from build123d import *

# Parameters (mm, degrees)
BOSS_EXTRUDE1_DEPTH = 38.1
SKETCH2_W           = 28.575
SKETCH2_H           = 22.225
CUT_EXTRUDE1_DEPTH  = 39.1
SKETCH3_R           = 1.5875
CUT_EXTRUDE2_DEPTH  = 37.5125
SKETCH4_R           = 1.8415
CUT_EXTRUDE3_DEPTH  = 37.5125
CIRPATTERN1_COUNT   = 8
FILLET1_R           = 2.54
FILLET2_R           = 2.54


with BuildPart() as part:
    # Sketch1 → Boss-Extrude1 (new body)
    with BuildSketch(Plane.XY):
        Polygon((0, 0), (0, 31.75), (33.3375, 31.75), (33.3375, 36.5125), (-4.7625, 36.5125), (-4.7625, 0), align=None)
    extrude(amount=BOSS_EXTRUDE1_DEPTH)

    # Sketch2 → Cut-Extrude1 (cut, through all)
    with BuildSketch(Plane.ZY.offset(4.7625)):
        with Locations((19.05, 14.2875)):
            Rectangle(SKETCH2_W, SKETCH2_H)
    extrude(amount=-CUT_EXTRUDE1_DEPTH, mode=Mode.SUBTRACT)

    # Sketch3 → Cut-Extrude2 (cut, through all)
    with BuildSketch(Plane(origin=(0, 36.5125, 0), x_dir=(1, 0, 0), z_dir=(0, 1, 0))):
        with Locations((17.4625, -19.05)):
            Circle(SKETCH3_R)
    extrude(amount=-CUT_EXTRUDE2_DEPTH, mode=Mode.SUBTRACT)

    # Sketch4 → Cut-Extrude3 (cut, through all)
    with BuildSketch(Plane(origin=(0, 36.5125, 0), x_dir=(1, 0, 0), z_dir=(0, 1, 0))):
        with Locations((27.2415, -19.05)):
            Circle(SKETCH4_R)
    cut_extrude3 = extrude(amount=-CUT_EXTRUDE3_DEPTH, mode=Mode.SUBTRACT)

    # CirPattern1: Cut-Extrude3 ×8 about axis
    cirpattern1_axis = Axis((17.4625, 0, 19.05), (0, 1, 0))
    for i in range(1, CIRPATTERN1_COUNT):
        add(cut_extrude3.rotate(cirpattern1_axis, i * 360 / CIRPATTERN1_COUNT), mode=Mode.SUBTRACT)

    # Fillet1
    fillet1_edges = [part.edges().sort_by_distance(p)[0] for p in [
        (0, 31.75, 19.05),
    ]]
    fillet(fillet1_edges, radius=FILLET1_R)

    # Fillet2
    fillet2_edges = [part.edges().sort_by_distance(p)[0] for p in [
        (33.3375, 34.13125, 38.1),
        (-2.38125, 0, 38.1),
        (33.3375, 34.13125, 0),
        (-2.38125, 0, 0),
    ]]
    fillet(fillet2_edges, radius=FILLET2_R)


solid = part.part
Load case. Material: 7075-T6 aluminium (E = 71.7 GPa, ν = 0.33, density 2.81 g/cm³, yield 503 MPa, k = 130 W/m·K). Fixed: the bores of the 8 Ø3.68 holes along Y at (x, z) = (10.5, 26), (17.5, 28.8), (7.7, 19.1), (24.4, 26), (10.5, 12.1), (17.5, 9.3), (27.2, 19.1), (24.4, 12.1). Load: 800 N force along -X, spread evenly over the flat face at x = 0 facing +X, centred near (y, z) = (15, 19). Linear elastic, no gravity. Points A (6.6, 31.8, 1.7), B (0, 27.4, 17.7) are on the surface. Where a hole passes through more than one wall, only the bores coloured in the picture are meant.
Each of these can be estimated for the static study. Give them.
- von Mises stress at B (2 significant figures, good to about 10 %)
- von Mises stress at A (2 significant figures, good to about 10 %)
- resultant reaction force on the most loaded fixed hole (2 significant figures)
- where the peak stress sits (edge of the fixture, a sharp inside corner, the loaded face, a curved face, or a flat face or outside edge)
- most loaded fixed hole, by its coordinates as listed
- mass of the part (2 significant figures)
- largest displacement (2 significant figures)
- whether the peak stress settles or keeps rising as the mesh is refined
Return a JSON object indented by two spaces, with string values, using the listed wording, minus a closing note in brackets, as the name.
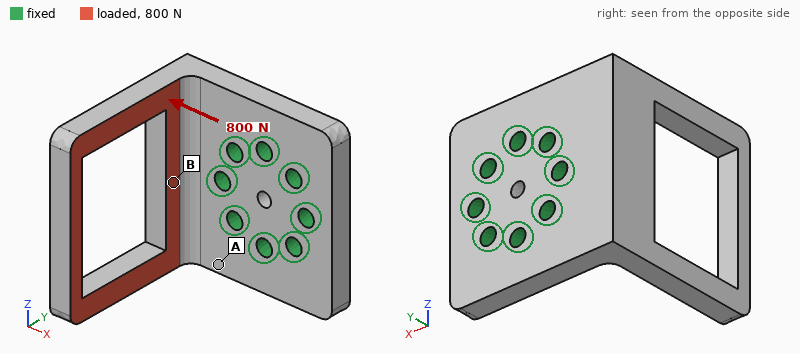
{
  "von Mises stress at B": "34 MPa",
  "von Mises stress at A": "76 MPa",
  "resultant reaction force on the most loaded fixed hole": "690 N",
  "where the peak stress sits": "edge of the fixture",
  "most loaded fixed hole, by its coordinates as listed": "(7.7, 19.1)",
  "mass of the part": "26 g",
  "largest displacement": "0.71 mm",
  "whether the peak stress settles or keeps rising as the mesh is refined": "keeps rising"
}
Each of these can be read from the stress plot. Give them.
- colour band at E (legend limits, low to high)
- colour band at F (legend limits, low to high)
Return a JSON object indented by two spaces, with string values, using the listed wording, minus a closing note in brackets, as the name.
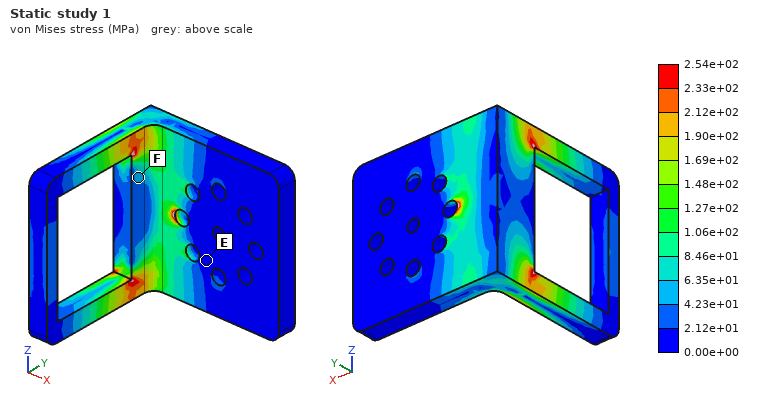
{
  "colour band at E": "0.00e+00 to 2.12e+01 MPa",
  "colour band at F": "4.23e+01 to 6.35e+01 MPa"
}
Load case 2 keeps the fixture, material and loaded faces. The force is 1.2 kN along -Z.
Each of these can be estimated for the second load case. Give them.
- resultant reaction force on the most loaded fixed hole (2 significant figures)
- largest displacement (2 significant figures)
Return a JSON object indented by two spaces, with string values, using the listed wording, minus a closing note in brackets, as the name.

{
  "resultant reaction force on the most loaded fixed hole": "960 N",
  "largest displacement": "0.48 mm"
}
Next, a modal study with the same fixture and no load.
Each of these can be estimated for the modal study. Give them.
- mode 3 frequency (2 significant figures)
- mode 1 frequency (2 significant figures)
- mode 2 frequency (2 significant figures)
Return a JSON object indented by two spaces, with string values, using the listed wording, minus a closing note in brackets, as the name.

{
  "mode 3 frequency": "4700 Hz",
  "mode 1 frequency": "2500 Hz",
  "mode 2 frequency": "3600 Hz"
}
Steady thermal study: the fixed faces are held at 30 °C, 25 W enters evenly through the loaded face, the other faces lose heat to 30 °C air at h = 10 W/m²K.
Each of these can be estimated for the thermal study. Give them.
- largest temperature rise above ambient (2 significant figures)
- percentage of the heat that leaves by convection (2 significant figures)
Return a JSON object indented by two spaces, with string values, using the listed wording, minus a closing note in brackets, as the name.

{
  "largest temperature rise above ambient": "80 K",
  "percentage of the heat that leaves by convection": "3.4 %"
}
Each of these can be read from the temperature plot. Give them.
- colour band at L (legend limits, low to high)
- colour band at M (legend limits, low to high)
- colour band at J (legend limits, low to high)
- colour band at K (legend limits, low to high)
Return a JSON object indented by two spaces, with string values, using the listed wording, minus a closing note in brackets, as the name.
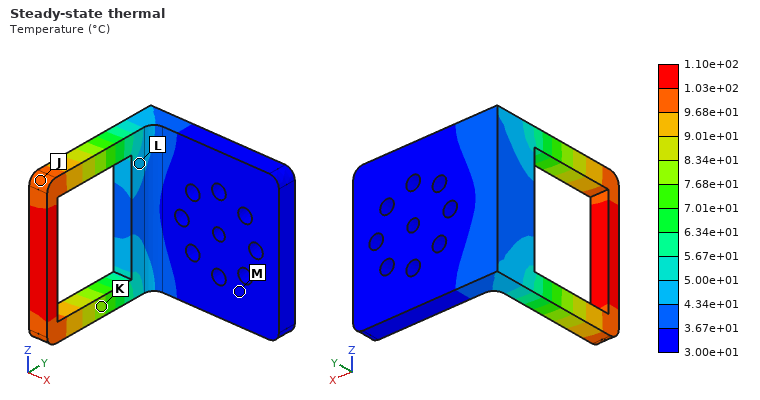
{
  "colour band at L": "4.34e+01 to 5.00e+01 °C",
  "colour band at M": "3.00e+01 to 3.67e+01 °C",
  "colour band at J": "9.68e+01 to 1.03e+02 °C",
  "colour band at K": "7.68e+01 to 8.34e+01 °C"
}
